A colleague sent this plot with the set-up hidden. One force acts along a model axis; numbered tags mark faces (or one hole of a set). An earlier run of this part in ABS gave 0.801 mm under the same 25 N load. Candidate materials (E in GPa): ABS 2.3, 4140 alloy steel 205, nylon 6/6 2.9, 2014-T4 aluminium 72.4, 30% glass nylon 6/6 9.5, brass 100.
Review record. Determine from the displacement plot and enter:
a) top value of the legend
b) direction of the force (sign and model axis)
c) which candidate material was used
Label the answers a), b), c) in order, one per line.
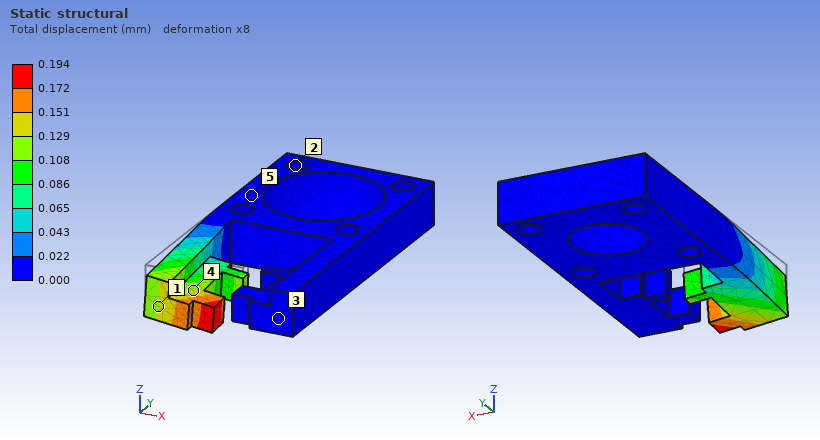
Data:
a) 0.194 mm
b) -Z
c) 30% glass nylon 6/6
